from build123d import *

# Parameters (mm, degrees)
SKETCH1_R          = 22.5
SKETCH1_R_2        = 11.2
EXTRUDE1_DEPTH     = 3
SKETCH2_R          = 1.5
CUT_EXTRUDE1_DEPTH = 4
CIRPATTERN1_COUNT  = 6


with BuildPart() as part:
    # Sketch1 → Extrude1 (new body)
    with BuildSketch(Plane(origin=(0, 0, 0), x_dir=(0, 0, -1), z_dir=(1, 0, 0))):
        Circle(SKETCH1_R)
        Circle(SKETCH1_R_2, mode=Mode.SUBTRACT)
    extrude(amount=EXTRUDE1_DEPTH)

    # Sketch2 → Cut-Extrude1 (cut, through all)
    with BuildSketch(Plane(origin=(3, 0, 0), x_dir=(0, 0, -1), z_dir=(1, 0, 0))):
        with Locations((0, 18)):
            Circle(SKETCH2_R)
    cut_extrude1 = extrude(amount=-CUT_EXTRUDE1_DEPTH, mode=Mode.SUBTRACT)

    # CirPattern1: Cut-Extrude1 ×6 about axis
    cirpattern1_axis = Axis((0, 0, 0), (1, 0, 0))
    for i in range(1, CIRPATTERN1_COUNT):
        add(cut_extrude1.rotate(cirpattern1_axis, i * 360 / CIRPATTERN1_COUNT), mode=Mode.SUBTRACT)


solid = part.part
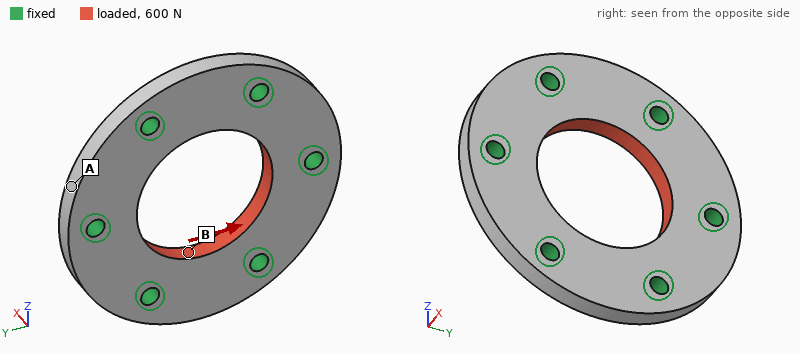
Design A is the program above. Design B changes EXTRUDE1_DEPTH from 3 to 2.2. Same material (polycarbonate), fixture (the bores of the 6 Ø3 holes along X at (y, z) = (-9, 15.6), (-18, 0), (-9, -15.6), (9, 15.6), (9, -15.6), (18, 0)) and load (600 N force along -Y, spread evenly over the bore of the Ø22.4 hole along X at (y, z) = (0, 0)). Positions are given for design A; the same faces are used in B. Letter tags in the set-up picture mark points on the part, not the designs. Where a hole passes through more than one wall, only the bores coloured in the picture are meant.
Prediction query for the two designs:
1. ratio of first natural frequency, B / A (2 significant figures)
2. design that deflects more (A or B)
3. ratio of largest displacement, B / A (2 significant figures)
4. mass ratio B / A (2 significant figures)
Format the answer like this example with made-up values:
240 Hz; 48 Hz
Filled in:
0.81; B; 1.4; 0.73
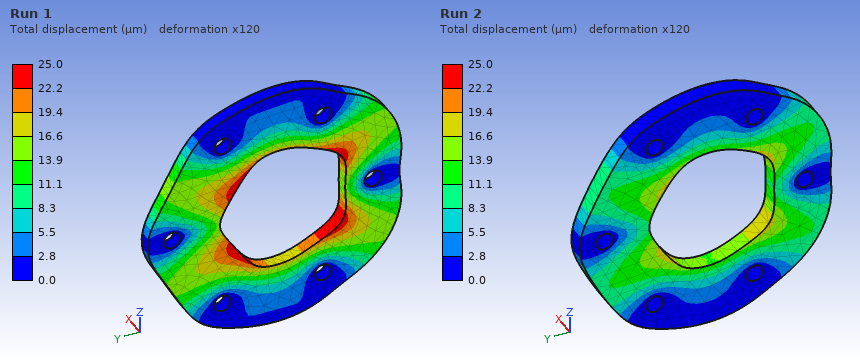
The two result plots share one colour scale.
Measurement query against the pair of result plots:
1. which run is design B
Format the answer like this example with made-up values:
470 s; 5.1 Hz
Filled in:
Run 1
